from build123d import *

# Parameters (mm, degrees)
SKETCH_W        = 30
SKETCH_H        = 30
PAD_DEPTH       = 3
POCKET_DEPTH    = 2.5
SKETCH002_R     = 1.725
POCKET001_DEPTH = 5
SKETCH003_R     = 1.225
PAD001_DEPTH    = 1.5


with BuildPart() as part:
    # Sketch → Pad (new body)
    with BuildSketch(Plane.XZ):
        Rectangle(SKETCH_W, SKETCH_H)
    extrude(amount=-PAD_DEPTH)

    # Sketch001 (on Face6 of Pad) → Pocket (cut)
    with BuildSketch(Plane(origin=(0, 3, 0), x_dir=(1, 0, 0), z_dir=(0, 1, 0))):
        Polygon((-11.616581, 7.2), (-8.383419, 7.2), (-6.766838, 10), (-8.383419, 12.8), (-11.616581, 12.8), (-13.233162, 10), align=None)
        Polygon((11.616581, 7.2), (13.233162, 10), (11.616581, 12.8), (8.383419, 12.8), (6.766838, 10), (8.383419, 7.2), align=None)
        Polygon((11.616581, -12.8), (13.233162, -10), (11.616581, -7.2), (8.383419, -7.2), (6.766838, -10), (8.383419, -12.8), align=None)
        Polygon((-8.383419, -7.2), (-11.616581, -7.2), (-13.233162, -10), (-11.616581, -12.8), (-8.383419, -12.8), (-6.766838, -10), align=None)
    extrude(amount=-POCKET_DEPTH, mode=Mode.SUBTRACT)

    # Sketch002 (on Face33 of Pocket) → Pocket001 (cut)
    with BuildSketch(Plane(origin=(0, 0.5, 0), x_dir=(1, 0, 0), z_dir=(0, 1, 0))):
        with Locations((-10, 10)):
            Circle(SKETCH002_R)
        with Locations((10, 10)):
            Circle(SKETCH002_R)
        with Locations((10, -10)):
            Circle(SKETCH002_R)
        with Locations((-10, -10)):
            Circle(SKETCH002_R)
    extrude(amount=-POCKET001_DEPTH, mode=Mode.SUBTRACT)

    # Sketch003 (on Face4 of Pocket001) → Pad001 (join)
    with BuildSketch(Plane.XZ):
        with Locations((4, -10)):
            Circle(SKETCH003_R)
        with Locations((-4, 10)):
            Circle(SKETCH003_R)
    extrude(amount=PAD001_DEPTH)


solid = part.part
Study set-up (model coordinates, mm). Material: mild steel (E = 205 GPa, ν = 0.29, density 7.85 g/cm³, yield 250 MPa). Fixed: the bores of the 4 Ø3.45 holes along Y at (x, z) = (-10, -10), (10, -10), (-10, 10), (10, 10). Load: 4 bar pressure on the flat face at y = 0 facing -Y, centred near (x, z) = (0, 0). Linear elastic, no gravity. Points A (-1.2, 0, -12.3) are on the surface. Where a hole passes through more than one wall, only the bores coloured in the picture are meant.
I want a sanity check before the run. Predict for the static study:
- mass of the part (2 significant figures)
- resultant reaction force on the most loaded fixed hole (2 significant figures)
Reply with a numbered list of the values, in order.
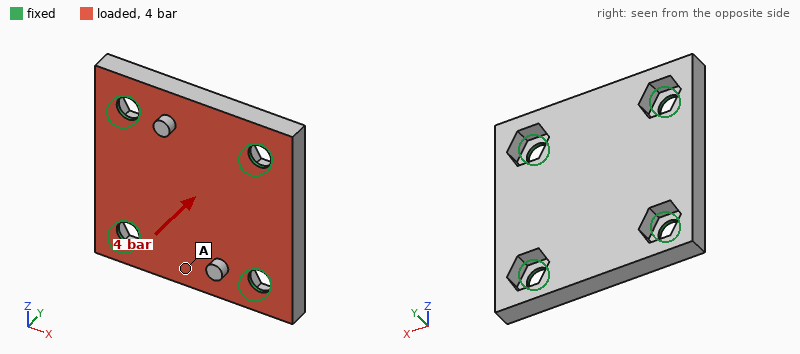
1. 19 g
2. 100 N
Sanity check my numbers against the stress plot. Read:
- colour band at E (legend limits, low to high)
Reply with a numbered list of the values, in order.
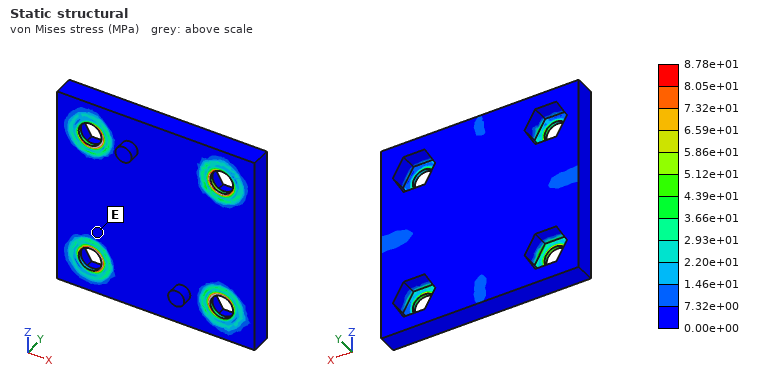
1. 0.00e+00 to 7.32e+00 MPa
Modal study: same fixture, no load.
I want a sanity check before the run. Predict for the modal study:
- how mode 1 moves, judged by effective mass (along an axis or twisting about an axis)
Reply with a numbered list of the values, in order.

1. along Y
